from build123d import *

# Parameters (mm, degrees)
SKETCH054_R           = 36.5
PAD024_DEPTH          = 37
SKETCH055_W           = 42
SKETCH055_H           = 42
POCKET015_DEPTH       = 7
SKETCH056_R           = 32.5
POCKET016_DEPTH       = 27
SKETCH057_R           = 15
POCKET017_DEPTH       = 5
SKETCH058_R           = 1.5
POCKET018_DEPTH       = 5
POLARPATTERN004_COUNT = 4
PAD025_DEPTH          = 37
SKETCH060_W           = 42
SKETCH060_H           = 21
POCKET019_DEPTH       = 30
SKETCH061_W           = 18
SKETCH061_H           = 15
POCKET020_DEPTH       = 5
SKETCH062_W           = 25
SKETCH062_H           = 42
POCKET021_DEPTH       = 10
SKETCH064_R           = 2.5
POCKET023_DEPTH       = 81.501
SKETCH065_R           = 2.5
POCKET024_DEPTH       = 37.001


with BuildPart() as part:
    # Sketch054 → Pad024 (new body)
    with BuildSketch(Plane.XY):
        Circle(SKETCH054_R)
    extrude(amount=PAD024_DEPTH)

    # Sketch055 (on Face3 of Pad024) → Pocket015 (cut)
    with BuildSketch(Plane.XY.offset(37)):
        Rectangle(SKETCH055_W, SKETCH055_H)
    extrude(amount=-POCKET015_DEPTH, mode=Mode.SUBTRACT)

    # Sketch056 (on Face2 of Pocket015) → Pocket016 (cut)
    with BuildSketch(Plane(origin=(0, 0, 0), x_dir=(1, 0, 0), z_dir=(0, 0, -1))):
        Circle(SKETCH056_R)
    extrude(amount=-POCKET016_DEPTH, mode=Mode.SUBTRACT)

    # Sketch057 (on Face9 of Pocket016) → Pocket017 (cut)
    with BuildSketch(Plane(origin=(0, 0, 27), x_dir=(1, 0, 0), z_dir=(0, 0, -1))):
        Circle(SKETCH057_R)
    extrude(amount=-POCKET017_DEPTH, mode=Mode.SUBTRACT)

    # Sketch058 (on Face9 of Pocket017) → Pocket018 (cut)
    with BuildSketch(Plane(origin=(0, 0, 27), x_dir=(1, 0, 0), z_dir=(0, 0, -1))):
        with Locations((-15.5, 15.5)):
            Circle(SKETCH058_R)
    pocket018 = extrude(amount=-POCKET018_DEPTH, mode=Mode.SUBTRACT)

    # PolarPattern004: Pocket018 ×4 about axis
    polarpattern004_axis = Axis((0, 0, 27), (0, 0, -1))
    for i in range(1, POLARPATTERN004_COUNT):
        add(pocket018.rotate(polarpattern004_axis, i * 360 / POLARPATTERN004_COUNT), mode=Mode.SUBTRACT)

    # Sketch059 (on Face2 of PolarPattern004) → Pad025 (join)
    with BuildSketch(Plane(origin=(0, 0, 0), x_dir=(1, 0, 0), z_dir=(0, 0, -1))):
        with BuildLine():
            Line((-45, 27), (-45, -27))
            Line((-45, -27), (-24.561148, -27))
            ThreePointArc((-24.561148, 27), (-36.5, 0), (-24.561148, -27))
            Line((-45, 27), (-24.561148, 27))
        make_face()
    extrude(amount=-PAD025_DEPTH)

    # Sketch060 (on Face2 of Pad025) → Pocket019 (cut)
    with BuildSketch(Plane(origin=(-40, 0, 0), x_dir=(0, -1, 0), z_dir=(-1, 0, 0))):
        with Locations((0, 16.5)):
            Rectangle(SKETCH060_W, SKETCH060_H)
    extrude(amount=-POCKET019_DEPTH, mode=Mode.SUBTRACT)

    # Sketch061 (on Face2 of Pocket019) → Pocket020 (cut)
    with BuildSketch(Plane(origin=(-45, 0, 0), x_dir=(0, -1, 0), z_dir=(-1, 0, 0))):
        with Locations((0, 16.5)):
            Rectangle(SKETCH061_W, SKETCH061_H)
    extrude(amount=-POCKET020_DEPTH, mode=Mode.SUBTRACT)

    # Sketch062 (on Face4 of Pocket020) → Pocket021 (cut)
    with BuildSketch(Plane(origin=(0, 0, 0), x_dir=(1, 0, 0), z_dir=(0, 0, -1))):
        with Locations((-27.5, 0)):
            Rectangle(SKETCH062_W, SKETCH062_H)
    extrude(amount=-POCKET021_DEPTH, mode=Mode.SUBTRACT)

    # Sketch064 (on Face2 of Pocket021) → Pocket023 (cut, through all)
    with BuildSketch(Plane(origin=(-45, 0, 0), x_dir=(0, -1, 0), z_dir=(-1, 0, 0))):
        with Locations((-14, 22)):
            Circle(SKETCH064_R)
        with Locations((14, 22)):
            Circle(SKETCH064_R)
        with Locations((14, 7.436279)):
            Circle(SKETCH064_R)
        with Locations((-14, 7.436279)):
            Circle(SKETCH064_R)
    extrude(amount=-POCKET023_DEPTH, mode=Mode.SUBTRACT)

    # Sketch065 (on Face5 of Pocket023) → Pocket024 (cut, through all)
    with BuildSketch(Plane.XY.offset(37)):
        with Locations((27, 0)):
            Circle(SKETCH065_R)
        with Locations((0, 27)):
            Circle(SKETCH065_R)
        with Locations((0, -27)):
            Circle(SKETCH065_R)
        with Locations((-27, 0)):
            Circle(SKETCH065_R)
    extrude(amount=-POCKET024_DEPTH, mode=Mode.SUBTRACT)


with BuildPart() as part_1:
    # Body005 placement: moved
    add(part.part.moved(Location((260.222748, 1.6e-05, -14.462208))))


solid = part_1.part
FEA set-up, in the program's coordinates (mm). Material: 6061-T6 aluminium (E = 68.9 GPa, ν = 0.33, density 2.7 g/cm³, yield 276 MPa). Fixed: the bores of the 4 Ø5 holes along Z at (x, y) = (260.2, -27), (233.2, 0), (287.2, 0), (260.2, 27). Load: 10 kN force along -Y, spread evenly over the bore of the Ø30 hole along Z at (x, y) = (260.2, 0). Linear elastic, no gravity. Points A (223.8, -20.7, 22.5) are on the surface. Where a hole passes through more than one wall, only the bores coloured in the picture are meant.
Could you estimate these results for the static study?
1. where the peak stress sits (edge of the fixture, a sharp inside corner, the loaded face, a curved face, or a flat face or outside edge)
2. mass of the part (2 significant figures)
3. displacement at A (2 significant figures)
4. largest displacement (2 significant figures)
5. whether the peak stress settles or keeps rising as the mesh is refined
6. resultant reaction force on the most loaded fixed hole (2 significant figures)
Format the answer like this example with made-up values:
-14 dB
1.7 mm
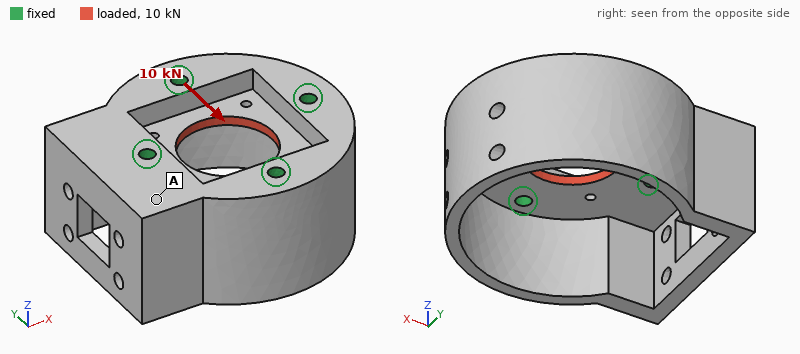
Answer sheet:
edge of the fixture
160 g
2.7 µm
12 µm
keeps rising
2.6 kN
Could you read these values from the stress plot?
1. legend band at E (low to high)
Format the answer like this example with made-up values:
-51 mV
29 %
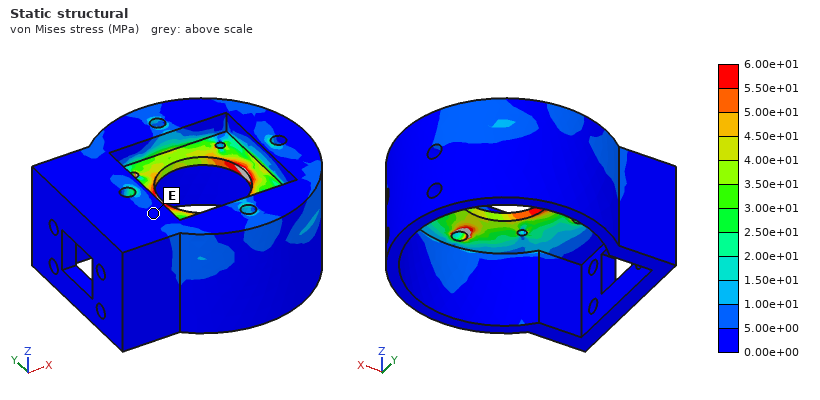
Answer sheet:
0.00e+00 to 5.00e+00 MPa
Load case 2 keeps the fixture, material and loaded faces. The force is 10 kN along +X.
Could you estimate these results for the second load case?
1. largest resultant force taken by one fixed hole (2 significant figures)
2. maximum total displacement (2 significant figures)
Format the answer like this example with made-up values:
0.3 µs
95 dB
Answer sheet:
2.6 kN
12 µm
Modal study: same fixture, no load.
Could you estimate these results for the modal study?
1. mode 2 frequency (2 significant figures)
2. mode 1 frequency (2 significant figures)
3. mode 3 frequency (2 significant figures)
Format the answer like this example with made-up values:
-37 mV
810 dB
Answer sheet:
6500 Hz
4500 Hz
7600 Hz
